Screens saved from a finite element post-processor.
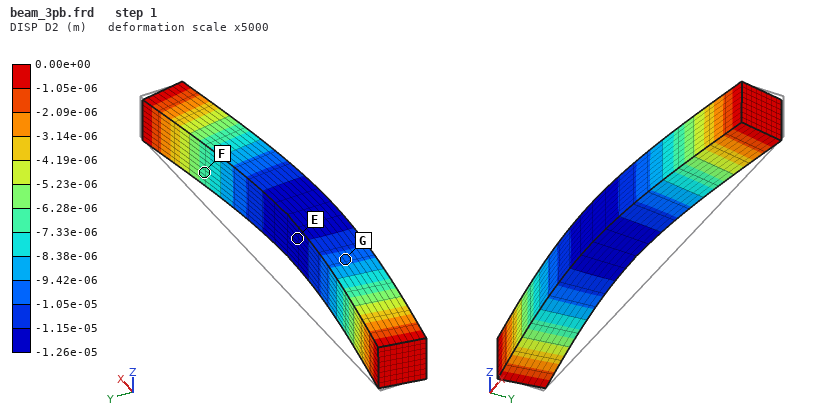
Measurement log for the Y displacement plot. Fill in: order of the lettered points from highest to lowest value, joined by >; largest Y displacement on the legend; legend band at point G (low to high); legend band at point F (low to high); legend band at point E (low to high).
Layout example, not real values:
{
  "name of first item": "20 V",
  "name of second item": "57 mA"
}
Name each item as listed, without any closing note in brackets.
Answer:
{
  "order of the lettered points from highest to lowest value, joined by >": "F > G > E",
  "largest Y displacement on the legend": "0.00e+00 m",
  "legend band at point G": "-1.05e-05 to -9.42e-06 m",
  "legend band at point F": "-7.33e-06 to -6.28e-06 m",
  "legend band at point E": "-1.26e-05 to -1.15e-05 m"
}
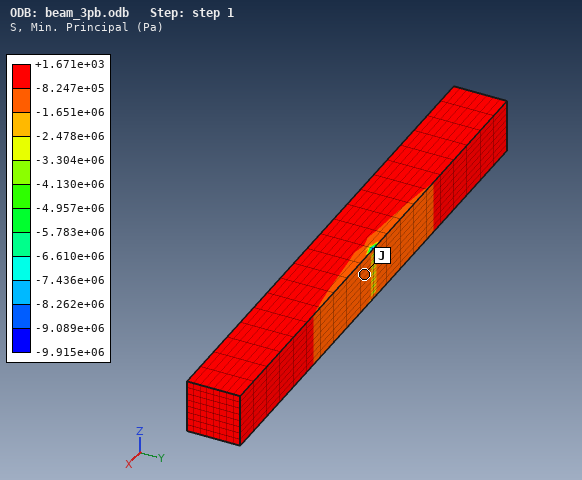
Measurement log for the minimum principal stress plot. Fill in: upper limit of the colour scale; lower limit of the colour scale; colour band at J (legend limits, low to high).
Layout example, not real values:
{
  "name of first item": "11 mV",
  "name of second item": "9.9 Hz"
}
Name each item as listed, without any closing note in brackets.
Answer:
{
  "upper limit of the colour scale": "+1.671e+03 Pa",
  "lower limit of the colour scale": "-9.915e+06 Pa",
  "colour band at J": "-1.651e+06 to -8.247e+05 Pa"
}
